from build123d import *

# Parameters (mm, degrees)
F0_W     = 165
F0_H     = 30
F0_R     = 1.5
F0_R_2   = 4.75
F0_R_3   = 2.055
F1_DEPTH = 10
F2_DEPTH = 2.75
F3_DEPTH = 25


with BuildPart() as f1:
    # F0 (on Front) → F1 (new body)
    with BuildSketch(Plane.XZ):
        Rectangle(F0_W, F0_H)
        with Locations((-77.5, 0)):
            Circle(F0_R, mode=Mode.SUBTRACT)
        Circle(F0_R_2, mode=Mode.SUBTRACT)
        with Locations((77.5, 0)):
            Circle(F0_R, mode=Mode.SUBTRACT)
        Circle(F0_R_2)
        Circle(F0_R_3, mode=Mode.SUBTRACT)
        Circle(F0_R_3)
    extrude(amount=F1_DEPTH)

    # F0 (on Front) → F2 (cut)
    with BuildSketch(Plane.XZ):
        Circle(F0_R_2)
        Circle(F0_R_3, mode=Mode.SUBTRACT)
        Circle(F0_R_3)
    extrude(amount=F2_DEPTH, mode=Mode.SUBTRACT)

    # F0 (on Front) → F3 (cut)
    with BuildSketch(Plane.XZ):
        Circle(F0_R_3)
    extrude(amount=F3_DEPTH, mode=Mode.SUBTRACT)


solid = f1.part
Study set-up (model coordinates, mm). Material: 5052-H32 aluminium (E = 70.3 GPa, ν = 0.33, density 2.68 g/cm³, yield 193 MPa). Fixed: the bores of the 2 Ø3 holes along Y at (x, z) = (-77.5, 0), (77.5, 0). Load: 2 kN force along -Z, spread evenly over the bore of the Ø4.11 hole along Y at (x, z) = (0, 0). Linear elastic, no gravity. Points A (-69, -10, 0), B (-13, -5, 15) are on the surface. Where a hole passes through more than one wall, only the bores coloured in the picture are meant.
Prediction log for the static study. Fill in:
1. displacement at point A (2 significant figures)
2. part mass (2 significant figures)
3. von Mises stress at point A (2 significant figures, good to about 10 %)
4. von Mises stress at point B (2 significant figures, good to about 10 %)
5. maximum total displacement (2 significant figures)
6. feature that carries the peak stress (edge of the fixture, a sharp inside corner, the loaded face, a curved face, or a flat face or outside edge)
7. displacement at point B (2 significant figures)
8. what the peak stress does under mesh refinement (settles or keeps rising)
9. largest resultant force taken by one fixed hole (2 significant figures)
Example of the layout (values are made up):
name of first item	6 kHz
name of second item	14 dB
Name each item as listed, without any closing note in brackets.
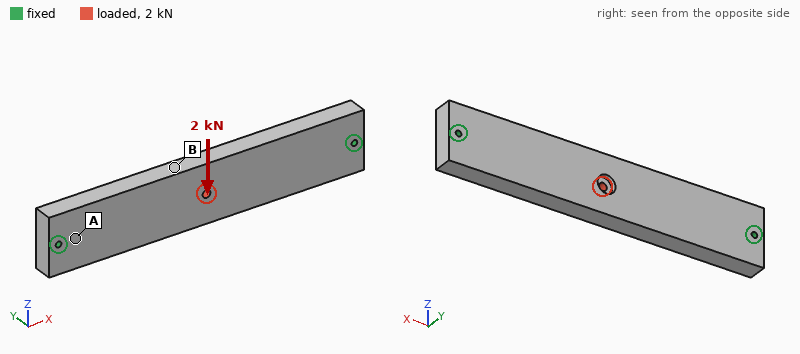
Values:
displacement at point A	14 µm
part mass	130 g
von Mises stress at point A	13 MPa
von Mises stress at point B	37 MPa
maximum total displacement	94 µm
feature that carries the peak stress	edge of the fixture
displacement at point B	84 µm
what the peak stress does under mesh refinement	keeps rising
largest resultant force taken by one fixed hole	1.0 kN
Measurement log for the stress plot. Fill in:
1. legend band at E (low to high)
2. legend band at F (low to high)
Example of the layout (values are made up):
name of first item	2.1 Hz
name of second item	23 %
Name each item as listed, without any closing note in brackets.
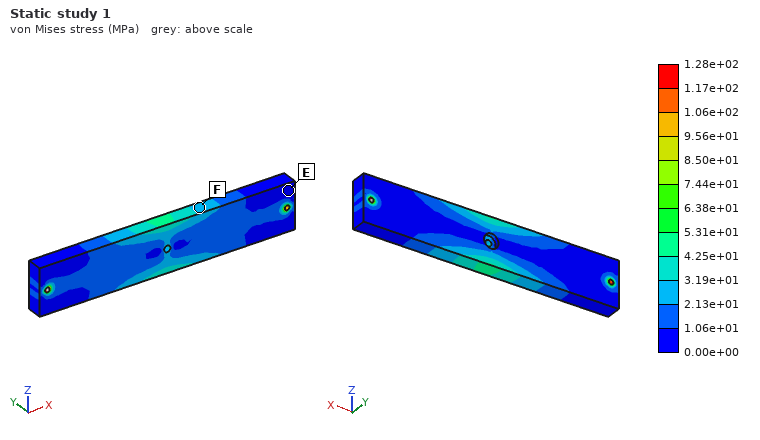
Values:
legend band at E	0.00e+00 to 1.06e+01 MPa
legend band at F	2.13e+01 to 3.19e+01 MPa
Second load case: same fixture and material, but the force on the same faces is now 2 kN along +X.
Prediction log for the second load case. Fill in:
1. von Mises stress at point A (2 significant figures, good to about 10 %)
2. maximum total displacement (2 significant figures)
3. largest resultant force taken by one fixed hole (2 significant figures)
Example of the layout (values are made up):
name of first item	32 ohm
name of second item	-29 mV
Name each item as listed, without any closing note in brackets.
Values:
von Mises stress at point A	6.1 MPa
maximum total displacement	6.5 µm
largest resultant force taken by one fixed hole	1.0 kN
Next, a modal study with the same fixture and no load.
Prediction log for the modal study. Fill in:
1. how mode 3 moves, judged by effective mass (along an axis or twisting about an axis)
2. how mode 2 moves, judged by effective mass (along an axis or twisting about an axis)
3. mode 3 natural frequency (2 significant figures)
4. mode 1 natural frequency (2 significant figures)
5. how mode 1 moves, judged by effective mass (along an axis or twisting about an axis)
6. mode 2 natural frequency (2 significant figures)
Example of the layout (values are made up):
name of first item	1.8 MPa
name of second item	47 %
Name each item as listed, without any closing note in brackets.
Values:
how mode 3 moves, judged by effective mass	twisting about Z
how mode 2 moves, judged by effective mass	along Z
mode 3 natural frequency	5000 Hz
mode 1 natural frequency	1800 Hz
how mode 1 moves, judged by effective mass	along Y
mode 2 natural frequency	3100 Hz
